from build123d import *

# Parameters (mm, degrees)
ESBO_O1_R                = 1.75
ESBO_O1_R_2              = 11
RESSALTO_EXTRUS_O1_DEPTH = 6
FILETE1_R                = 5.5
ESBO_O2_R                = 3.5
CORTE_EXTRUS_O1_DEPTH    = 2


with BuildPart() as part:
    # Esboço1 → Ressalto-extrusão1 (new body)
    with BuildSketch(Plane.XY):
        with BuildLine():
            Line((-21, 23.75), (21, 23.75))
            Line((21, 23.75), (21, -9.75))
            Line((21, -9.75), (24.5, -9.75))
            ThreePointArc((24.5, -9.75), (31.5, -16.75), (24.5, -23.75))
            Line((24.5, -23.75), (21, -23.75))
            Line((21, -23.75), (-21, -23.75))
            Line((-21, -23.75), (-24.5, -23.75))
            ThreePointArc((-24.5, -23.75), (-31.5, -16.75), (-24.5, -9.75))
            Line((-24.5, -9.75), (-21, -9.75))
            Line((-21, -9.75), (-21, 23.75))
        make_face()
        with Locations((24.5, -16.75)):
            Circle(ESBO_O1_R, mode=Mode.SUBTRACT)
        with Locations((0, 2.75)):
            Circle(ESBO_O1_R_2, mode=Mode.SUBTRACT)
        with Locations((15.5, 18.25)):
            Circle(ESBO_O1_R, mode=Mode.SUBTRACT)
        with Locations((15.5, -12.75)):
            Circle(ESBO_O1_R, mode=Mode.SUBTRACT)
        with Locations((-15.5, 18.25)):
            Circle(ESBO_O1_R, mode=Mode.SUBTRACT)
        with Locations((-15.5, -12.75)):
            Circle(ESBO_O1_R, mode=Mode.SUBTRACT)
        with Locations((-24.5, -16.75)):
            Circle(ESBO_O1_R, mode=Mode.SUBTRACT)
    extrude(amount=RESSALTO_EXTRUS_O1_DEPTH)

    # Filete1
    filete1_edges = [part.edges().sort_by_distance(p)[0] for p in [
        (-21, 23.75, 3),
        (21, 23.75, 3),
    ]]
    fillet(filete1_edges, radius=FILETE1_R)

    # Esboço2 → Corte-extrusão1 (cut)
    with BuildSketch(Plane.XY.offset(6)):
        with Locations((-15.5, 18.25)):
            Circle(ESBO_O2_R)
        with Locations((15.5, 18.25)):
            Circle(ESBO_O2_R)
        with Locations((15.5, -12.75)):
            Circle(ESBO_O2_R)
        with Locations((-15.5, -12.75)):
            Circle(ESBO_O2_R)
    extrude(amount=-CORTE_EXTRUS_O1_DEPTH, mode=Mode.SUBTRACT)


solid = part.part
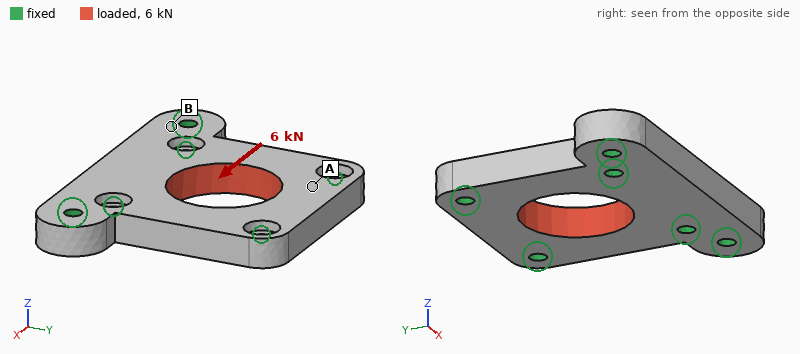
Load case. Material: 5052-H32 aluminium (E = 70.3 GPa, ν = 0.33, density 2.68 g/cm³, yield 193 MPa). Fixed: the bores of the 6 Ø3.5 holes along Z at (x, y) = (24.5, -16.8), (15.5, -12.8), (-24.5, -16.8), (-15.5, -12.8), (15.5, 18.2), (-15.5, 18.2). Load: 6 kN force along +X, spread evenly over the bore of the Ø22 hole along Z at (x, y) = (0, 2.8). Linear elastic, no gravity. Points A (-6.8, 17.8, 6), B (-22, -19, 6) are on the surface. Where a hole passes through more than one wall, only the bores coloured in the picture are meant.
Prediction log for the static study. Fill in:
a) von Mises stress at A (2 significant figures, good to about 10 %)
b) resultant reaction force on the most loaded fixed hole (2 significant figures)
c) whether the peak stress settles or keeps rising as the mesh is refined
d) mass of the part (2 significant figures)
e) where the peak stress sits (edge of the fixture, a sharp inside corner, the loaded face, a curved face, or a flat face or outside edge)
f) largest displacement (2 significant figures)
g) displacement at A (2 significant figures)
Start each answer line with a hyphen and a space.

- 13 MPa
- 1.5 kN
- keeps rising
- 28 g
- edge of the fixture
- 9.8 µm
- 2.9 µm
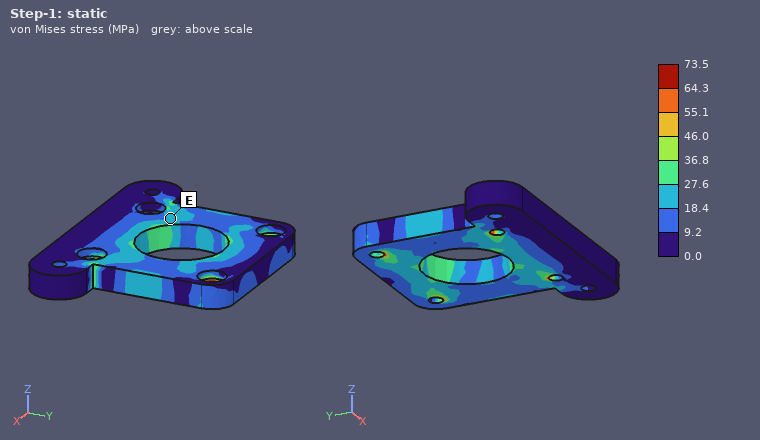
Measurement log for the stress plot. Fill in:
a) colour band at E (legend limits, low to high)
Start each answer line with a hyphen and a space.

- 18.4 to 27.6 MPa
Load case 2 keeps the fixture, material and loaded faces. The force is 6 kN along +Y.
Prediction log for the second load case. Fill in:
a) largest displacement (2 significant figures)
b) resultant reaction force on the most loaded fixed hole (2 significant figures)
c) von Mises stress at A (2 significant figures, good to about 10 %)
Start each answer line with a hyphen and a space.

- 11 µm
- 1.5 kN
- 21 MPa
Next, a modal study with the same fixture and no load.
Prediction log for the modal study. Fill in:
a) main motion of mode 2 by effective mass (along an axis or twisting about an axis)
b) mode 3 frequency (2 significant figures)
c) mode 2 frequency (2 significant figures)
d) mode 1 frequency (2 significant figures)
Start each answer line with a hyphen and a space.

- along Z
- 25 kHz
- 22 kHz
- 20 kHz
